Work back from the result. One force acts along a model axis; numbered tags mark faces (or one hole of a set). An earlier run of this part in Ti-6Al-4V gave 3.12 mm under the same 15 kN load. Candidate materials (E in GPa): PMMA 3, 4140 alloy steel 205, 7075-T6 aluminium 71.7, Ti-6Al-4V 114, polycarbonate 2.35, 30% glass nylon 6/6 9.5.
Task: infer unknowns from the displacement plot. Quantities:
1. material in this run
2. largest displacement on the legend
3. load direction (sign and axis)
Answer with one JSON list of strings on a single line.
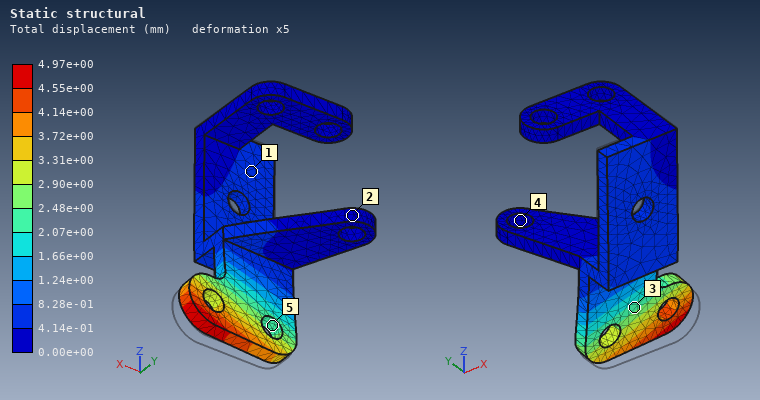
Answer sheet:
["7075-T6 aluminium", "4.97e+00 mm", "+Y"]
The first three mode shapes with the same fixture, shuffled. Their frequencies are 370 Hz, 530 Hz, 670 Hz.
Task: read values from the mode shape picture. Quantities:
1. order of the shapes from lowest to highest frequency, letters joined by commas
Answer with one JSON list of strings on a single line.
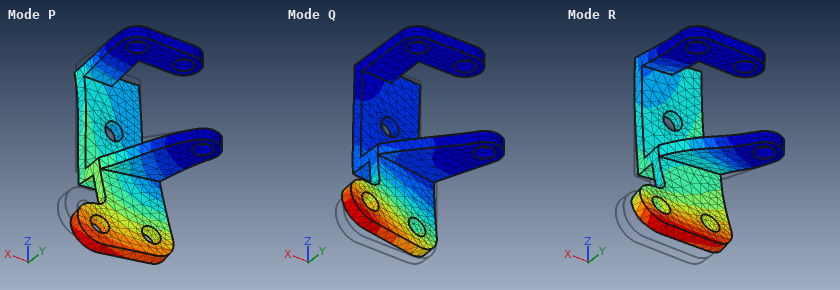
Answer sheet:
["Q, P, R"]
